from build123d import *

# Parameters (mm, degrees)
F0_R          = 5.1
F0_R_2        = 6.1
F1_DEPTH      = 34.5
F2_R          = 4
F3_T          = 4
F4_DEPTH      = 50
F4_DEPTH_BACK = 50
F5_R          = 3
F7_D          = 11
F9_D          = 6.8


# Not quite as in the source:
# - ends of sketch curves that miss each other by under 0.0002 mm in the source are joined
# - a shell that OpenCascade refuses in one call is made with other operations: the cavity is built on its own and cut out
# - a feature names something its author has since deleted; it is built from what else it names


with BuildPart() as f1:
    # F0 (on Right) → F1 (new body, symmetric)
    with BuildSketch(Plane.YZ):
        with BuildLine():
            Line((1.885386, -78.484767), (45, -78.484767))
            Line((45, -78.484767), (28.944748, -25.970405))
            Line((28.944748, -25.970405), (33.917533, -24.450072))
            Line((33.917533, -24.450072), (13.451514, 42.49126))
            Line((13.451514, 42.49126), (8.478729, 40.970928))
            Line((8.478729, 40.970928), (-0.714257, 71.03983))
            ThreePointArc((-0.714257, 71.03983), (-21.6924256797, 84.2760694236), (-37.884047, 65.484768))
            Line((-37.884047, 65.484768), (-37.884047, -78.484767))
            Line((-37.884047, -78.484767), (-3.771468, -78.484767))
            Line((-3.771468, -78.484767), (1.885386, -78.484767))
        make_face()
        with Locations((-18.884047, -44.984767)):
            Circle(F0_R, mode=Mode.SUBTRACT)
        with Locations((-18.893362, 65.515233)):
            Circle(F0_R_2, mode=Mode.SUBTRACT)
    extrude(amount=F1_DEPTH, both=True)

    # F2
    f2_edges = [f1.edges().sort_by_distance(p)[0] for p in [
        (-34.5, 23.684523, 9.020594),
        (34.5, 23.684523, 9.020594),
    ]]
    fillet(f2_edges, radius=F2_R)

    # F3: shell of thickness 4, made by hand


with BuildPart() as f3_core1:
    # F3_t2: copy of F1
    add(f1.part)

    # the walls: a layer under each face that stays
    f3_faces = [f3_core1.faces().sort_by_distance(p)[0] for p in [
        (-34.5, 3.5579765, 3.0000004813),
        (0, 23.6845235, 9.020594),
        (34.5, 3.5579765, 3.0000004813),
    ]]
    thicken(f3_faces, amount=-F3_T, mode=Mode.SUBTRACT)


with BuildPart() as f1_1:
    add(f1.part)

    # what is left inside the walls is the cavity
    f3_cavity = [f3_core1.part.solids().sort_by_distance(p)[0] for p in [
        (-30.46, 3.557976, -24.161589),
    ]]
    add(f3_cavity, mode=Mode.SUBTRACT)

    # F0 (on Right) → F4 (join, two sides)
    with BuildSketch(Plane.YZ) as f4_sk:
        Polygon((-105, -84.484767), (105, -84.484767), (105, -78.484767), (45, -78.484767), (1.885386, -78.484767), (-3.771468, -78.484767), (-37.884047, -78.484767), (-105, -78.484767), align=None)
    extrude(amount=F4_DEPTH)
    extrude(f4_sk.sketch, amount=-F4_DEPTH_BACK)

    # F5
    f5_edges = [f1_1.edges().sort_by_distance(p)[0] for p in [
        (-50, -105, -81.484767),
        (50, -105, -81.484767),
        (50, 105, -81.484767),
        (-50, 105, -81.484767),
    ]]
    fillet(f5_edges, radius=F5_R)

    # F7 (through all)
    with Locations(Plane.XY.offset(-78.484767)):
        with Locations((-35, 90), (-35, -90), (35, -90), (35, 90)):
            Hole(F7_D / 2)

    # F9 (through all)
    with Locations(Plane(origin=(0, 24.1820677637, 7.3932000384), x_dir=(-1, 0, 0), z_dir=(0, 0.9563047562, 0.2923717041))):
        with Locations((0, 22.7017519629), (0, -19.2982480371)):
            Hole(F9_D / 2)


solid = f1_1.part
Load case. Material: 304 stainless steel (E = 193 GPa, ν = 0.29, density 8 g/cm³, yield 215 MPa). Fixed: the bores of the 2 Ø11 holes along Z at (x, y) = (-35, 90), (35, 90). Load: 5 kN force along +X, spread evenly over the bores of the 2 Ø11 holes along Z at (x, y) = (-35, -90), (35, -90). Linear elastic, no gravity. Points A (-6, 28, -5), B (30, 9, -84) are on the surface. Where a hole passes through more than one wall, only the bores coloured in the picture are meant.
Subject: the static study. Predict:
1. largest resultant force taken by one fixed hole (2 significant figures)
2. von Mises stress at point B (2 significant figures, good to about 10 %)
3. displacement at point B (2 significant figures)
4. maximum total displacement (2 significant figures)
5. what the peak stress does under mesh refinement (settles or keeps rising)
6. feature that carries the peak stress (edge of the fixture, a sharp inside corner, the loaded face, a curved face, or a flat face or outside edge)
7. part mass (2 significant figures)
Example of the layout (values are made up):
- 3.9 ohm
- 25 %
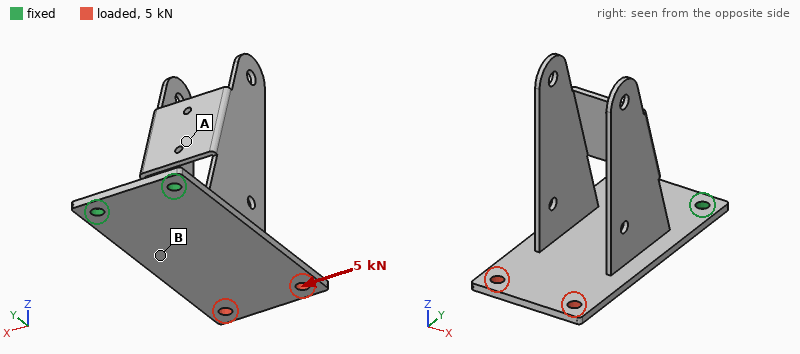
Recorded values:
- 12 kN
- 30 MPa
- 0.043 mm
- 0.14 mm
- keeps rising
- edge of the fixture
- 1.7 kg
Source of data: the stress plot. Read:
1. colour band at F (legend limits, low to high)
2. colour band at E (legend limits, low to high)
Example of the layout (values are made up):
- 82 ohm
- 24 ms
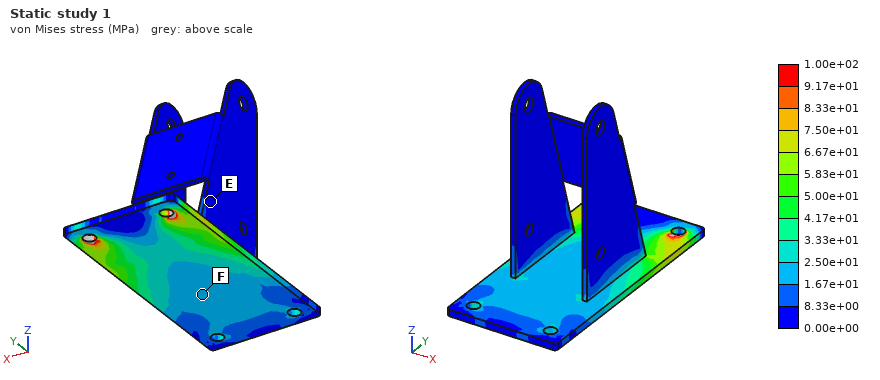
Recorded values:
- 1.67e+01 to 2.50e+01 MPa
- 0.00e+00 to 8.33e+00 MPa
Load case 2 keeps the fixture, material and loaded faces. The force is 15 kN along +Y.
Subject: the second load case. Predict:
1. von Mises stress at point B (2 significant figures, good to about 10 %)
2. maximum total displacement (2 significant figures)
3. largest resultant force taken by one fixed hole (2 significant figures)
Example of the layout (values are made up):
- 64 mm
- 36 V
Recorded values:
- 23 MPa
- 52 µm
- 7.6 kN
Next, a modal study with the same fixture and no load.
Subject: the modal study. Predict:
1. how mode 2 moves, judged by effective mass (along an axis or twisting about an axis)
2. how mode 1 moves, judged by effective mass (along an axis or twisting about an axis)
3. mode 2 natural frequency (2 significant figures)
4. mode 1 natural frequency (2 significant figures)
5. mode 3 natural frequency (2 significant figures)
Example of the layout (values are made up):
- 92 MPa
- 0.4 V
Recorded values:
- along X
- along Z
- 260 Hz
- 100 Hz
- 520 Hz
